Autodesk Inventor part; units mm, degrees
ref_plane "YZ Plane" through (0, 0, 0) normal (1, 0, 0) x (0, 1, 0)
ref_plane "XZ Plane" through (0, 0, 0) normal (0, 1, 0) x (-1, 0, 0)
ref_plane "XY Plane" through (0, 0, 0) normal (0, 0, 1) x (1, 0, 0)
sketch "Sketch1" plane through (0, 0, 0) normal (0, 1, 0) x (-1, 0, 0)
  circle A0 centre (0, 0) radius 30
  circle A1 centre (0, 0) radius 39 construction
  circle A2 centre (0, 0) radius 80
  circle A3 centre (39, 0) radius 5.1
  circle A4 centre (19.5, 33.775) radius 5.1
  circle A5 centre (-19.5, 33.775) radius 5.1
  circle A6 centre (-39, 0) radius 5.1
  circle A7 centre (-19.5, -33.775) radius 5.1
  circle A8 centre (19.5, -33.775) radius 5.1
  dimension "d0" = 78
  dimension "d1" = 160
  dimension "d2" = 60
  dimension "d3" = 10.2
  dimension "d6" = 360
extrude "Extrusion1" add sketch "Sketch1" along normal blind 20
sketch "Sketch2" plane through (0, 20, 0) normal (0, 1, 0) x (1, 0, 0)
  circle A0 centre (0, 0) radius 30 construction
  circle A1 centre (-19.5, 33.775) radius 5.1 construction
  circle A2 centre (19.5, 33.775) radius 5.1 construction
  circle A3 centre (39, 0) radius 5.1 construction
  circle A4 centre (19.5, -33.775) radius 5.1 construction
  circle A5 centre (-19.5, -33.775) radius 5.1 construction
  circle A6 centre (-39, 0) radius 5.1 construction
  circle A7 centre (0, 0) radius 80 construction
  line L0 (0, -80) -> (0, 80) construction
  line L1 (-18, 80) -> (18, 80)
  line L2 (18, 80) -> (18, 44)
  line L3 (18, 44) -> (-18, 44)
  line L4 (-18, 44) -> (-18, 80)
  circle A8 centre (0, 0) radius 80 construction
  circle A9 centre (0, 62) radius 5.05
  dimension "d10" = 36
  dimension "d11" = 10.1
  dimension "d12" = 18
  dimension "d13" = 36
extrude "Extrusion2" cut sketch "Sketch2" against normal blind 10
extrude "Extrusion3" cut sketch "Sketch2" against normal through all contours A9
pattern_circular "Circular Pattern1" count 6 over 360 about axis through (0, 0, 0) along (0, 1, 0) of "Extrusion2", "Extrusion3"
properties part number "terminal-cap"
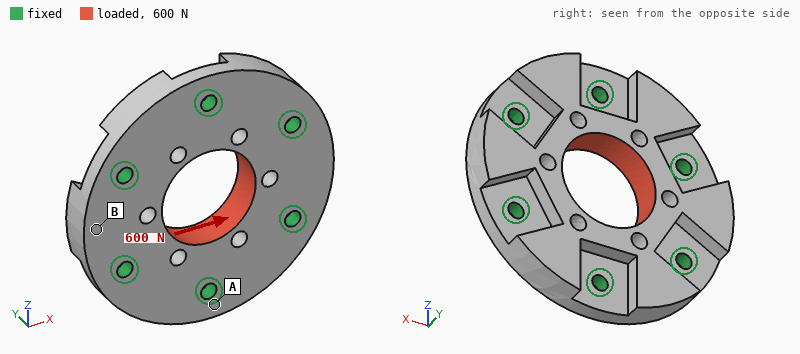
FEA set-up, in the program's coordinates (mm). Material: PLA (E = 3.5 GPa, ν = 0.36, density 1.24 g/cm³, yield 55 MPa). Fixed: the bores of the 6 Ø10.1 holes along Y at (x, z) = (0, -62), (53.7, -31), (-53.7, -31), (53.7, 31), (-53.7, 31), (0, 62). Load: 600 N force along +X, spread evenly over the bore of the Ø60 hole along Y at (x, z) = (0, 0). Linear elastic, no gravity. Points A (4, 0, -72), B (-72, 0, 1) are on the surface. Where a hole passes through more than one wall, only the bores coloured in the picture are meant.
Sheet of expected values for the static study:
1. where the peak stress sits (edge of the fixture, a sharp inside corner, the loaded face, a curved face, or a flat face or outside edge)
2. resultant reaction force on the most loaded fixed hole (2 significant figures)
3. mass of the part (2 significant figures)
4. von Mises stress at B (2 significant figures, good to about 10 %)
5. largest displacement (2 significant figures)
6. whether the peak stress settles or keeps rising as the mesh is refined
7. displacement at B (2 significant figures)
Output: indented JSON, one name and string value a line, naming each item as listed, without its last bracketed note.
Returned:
{
  "where the peak stress sits": "edge of the fixture",
  "resultant reaction force on the most loaded fixed hole": "120 N",
  "mass of the part": "320 g",
  "von Mises stress at B": "0.15 MPa",
  "largest displacement": "8.1 µm",
  "whether the peak stress settles or keeps rising as the mesh is refined": "keeps rising",
  "displacement at B": "2.6 µm"
}
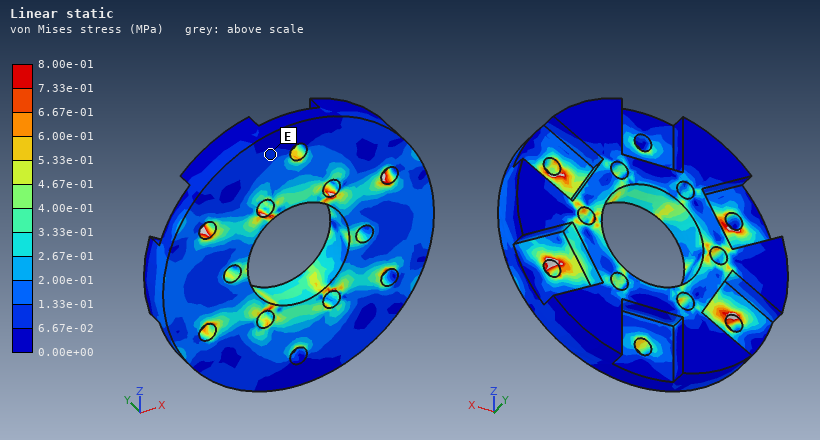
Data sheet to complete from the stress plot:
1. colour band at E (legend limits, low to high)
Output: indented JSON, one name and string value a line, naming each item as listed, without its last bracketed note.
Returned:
{
  "colour band at E": "6.67e-02 to 1.33e-01 MPa"
}
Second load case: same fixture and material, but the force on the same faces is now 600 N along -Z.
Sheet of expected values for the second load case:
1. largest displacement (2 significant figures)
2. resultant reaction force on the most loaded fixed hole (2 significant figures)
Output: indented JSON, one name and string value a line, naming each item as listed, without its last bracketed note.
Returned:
{
  "largest displacement": "7.2 µm",
  "resultant reaction force on the most loaded fixed hole": "130 N"
}
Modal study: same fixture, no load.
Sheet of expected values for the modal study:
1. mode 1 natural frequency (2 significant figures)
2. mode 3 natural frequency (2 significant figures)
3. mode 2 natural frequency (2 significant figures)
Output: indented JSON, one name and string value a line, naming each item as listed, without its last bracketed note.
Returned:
{
  "mode 1 natural frequency": "2600 Hz",
  "mode 3 natural frequency": "2900 Hz",
  "mode 2 natural frequency": "2800 Hz"
}
